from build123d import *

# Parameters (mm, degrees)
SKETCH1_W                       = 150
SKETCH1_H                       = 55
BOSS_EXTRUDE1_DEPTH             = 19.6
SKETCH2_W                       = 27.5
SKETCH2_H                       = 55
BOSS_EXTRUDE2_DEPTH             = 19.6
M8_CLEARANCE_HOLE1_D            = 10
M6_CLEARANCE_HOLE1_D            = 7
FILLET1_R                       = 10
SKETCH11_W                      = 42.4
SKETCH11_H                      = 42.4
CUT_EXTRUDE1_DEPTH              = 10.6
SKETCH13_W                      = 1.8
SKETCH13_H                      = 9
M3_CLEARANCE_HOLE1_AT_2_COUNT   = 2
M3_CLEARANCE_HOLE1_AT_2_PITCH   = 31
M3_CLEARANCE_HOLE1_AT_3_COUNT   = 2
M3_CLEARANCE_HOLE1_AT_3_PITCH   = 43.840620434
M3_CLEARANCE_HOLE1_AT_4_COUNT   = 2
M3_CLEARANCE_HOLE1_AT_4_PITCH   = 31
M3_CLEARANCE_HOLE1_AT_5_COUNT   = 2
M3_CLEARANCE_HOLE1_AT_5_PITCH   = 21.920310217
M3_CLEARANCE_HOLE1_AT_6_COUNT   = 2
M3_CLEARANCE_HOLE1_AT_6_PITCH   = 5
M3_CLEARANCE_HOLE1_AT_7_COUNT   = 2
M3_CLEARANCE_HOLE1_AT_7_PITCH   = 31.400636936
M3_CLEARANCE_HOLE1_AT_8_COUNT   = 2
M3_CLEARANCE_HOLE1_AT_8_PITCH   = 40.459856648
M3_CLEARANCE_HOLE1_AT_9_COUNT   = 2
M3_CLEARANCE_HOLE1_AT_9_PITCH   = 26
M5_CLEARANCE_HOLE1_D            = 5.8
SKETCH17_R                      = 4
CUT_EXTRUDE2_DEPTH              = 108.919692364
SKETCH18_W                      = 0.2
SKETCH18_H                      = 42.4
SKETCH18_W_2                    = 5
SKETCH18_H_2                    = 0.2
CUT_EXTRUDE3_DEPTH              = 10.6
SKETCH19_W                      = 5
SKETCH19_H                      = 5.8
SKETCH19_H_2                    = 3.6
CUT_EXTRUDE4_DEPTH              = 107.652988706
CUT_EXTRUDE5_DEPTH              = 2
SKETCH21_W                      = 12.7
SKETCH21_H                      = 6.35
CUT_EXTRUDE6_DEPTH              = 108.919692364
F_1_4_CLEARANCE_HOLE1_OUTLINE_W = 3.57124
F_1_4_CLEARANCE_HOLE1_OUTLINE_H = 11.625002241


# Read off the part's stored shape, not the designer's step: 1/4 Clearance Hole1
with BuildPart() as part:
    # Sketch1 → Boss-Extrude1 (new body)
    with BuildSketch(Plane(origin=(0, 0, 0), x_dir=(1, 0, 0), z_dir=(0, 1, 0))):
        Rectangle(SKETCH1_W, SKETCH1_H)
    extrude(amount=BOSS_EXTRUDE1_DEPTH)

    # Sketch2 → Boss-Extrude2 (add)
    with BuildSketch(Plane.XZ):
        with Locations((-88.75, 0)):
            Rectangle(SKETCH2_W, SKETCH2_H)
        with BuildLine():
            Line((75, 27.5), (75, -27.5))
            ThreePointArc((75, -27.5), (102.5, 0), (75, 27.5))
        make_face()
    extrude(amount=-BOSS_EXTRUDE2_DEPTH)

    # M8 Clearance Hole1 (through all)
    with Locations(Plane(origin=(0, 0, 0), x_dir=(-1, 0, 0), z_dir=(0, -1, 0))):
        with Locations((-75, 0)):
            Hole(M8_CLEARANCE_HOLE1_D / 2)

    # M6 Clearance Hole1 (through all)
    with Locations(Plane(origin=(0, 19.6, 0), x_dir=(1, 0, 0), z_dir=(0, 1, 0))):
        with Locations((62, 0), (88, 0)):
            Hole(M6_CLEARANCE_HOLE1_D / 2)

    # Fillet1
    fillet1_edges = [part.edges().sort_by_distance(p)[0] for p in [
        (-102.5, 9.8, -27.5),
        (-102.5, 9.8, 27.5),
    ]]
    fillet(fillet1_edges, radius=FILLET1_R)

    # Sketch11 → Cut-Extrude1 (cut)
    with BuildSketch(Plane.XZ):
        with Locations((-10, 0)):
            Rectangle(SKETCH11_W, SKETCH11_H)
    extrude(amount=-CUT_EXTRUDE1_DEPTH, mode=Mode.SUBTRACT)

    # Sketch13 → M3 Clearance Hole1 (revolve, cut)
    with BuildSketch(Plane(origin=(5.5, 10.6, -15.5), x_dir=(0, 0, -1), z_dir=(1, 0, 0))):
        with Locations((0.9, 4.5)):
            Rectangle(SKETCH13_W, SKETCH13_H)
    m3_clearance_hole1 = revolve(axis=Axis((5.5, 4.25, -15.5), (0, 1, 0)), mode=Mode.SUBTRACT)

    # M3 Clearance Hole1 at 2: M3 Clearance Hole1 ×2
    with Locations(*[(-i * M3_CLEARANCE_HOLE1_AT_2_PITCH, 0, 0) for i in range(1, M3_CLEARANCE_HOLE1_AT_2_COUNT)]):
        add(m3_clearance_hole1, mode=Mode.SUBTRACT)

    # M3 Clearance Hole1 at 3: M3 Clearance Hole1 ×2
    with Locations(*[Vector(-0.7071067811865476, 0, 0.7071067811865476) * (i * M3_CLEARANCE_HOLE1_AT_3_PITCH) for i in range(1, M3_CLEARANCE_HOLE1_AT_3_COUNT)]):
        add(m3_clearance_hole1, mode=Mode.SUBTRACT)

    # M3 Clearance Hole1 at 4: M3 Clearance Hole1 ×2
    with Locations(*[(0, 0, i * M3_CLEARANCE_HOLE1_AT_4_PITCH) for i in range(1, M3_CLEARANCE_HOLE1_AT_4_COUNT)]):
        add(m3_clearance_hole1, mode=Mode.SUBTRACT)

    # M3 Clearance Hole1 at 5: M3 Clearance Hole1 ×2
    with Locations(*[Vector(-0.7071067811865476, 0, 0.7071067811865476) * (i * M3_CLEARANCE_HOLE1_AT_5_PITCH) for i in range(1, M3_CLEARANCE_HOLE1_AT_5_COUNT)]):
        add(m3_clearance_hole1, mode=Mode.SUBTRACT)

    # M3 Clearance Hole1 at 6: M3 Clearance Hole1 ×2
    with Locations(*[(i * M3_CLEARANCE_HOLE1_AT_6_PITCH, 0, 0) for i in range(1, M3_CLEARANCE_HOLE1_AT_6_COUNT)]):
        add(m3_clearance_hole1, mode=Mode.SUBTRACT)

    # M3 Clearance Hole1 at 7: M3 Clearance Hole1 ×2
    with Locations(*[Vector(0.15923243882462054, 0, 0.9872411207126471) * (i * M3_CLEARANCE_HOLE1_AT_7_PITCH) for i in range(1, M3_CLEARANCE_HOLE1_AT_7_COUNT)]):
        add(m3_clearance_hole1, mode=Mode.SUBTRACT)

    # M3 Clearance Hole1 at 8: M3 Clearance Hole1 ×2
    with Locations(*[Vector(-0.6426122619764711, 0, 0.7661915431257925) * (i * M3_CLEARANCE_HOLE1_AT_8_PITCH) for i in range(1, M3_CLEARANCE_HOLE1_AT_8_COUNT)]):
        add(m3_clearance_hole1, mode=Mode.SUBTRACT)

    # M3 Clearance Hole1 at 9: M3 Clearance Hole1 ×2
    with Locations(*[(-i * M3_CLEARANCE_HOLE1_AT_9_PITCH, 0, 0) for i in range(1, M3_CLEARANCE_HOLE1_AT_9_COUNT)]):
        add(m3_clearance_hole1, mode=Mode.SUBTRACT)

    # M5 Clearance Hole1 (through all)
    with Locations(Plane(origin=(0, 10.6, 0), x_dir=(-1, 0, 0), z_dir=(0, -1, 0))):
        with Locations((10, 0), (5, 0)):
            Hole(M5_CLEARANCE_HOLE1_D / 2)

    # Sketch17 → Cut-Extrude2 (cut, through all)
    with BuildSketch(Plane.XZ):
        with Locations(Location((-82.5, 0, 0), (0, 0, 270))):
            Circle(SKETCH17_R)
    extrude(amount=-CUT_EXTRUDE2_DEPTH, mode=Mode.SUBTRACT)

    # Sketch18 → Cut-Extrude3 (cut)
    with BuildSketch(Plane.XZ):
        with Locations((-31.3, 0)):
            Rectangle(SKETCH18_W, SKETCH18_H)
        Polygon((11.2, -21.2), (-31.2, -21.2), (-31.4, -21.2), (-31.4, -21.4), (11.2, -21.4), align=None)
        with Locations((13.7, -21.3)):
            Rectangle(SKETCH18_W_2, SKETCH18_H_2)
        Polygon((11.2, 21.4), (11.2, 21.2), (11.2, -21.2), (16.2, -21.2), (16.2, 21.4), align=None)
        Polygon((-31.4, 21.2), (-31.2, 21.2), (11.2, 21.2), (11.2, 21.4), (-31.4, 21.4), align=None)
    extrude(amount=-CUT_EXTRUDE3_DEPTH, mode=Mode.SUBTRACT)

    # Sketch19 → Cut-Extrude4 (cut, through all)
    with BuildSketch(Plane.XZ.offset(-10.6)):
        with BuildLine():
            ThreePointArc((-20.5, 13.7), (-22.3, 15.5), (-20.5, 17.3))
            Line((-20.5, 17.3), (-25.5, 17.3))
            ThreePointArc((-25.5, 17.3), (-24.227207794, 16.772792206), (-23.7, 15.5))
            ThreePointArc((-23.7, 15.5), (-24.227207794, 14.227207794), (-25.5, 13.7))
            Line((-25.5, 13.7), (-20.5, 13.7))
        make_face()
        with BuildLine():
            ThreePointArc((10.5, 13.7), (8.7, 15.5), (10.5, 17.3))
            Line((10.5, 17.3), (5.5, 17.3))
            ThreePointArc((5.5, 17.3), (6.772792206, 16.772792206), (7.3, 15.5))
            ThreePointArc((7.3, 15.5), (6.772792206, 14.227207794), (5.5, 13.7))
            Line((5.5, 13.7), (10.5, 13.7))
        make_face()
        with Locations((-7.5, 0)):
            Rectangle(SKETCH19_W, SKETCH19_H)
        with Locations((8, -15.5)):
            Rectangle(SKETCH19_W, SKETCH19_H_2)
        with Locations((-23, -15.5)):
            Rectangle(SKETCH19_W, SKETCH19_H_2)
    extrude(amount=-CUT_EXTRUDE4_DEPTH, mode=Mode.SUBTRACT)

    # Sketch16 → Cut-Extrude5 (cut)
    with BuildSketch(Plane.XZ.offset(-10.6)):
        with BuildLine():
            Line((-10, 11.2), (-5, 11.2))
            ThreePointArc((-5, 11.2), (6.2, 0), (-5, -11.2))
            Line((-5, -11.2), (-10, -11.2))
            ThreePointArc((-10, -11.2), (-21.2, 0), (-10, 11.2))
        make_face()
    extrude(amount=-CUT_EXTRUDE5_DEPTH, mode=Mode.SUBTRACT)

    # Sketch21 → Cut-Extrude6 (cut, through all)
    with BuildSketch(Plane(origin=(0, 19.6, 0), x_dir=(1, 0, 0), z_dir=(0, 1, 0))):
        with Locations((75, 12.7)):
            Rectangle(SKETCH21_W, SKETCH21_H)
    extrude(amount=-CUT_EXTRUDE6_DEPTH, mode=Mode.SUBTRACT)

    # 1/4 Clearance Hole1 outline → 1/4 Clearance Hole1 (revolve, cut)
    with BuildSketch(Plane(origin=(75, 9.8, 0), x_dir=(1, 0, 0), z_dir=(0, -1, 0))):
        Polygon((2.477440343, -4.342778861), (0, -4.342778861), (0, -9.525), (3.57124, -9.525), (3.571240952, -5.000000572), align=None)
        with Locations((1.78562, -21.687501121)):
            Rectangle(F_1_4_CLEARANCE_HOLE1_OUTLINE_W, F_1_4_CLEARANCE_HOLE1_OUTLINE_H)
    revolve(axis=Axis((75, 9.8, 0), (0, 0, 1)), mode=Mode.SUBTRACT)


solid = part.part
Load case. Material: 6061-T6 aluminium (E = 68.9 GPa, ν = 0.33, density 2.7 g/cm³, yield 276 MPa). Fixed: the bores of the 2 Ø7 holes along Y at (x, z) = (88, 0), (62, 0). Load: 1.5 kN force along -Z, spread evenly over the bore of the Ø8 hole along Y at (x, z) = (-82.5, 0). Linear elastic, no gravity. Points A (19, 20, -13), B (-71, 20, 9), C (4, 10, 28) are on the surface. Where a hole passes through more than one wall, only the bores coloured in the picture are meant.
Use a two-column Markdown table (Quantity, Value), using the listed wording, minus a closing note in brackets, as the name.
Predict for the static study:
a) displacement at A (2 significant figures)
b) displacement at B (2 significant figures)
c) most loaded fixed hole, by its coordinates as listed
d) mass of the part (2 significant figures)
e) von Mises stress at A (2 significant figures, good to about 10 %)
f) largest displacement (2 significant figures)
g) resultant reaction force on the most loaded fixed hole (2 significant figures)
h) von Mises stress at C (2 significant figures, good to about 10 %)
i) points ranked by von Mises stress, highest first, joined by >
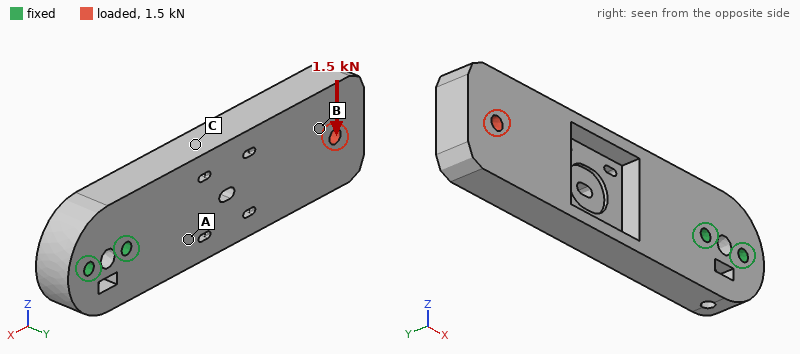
| Quantity | Value |
|---|---|
| displacement at A | 0.040 mm |
| displacement at B | 0.17 mm |
| most loaded fixed hole, by its coordinates as listed | (62, 0) |
| mass of the part | 500 g |
| von Mises stress at A | 10 MPa |
| largest displacement | 0.24 mm |
| resultant reaction force on the most loaded fixed hole | 6.9 kN |
| von Mises stress at C | 20 MPa |
| points ranked by von Mises stress, highest first, joined by > | C > A > B |
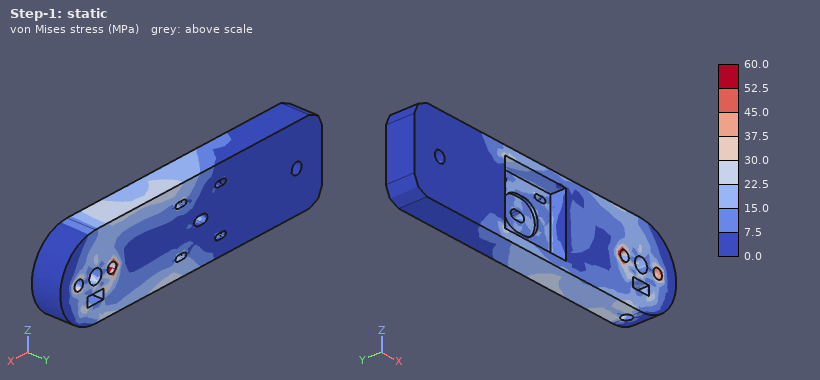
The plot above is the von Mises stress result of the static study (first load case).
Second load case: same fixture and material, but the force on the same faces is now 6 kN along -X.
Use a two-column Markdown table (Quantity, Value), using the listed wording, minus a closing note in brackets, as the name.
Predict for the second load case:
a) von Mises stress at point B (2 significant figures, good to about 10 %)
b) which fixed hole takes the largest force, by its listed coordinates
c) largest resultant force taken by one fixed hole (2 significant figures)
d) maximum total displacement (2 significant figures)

| Quantity | Value |
|---|---|
| von Mises stress at point B | 8.1 MPa |
| which fixed hole takes the largest force, by its listed coordinates | (62, 0) |
| largest resultant force taken by one fixed hole | 4.6 kN |
| maximum total displacement | 0.13 mm |
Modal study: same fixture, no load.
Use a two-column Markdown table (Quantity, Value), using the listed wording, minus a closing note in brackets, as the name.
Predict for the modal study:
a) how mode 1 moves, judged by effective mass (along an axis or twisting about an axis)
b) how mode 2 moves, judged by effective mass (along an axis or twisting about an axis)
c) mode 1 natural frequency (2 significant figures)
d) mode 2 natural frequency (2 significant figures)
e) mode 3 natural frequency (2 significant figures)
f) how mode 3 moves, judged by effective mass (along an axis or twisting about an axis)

| Quantity | Value |
|---|---|
| how mode 1 moves, judged by effective mass | along Y |
| how mode 2 moves, judged by effective mass | along Z |
| mode 1 natural frequency | 480 Hz |
| mode 2 natural frequency | 1000 Hz |
| mode 3 natural frequency | 2000 Hz |
| how mode 3 moves, judged by effective mass | twisting about X |
